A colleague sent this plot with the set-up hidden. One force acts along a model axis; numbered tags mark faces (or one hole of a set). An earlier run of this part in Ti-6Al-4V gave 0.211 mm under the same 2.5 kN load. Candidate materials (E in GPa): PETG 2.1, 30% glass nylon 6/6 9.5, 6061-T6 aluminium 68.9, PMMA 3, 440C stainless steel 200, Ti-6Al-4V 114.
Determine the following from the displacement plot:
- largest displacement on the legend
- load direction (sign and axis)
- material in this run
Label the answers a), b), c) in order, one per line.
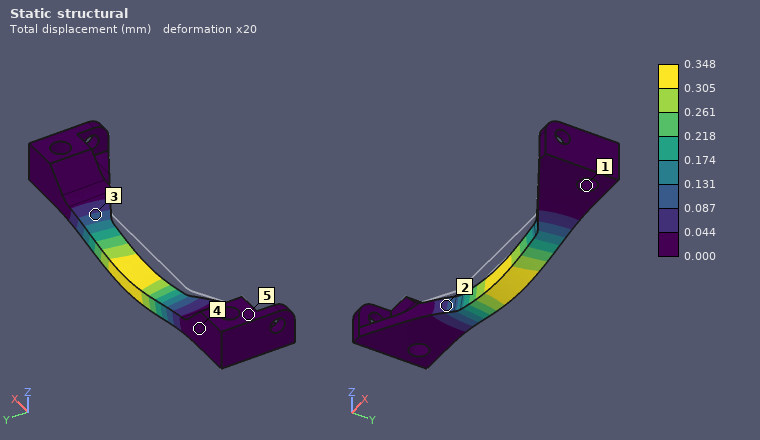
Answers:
a) 0.348 mm
b) -Z
c) 6061-T6 aluminium
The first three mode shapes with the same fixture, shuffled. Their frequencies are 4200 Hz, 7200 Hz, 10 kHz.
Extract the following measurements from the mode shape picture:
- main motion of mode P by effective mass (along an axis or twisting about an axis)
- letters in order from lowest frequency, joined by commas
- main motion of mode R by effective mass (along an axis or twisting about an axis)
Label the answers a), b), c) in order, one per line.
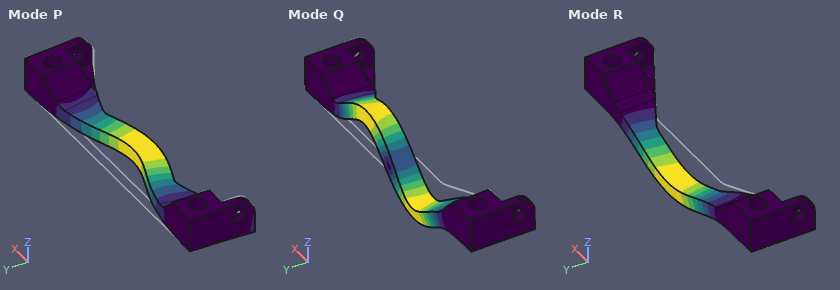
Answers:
a) along Y
b) R, P, Q
c) along Z
